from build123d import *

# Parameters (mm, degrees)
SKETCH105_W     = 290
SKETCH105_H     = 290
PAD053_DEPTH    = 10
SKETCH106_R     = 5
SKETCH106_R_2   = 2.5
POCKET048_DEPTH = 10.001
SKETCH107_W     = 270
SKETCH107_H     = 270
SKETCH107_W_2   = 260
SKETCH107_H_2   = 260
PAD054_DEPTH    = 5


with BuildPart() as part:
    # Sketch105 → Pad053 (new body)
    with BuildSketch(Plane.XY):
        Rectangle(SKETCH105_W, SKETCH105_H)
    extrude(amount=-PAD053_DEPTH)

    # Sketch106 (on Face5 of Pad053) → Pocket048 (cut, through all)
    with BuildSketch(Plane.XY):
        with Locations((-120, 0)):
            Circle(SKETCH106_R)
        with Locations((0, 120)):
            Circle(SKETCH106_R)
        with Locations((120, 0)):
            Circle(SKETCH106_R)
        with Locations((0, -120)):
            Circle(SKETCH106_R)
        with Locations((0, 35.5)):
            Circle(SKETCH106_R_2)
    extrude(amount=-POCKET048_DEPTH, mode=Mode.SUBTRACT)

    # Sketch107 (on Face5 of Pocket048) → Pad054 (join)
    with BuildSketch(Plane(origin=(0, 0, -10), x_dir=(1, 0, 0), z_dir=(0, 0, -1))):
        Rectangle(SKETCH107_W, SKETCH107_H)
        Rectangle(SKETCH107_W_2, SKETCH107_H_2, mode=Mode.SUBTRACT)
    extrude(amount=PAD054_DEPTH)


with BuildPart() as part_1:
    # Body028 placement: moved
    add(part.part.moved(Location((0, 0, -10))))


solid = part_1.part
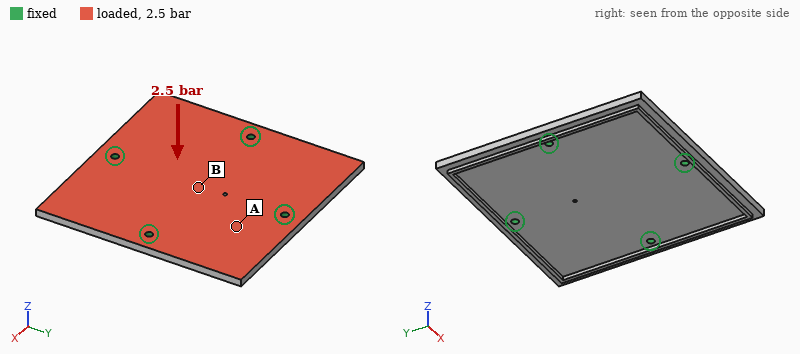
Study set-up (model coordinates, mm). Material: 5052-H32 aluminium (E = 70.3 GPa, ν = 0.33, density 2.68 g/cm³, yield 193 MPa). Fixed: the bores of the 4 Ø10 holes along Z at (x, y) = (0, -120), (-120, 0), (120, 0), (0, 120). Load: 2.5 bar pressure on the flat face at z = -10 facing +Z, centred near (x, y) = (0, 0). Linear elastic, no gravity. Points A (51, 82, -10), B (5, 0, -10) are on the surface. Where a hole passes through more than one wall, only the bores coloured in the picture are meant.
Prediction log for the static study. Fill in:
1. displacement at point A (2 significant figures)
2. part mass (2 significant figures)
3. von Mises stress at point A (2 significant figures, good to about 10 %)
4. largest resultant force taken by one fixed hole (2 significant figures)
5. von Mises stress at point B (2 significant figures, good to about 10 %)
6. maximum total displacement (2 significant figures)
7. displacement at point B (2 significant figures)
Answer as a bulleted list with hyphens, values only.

- 0.14 mm
- 2.3 kg
- 27 MPa
- 5.2 kN
- 12 MPa
- 0.56 mm
- 0.16 mm
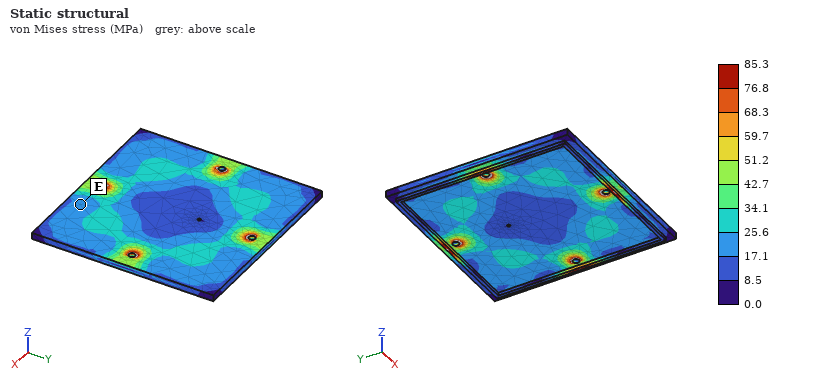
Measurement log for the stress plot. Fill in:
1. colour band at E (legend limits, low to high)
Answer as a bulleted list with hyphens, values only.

- 17.1 to 25.6 MPa
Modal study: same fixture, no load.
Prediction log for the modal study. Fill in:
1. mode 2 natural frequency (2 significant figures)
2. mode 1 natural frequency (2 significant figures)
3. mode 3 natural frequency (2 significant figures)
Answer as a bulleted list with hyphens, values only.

- 790 Hz
- 730 Hz
- 790 Hz
